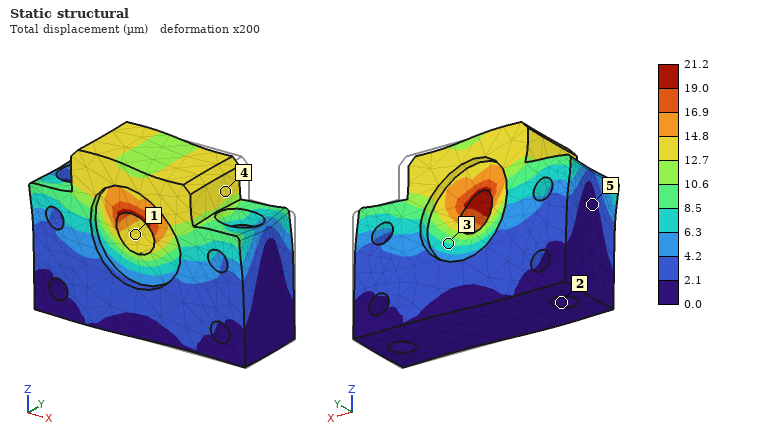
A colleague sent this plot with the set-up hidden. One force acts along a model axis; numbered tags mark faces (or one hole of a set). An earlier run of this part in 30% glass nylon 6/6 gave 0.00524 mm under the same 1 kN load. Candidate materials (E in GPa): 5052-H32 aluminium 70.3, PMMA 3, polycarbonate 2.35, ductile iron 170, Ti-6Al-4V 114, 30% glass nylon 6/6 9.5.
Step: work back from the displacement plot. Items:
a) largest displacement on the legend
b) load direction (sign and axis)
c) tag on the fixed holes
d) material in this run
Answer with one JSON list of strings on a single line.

["21.2 µm", "-X", "2", "polycarbonate"]
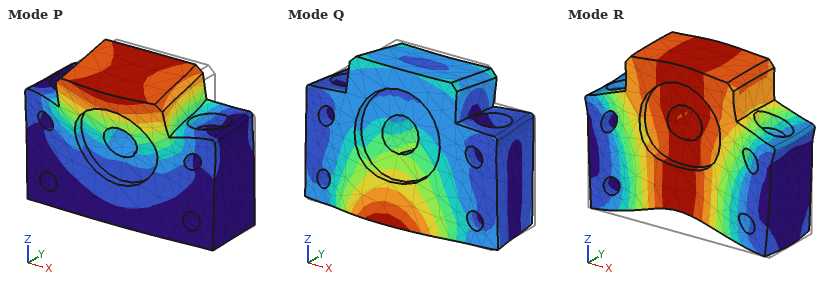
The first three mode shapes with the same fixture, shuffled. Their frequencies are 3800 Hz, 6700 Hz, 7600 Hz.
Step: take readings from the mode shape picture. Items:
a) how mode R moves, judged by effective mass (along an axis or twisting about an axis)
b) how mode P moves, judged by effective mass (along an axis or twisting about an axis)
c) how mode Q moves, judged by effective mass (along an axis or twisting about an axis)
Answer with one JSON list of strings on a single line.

["along Z", "along Y", "along Y"]
